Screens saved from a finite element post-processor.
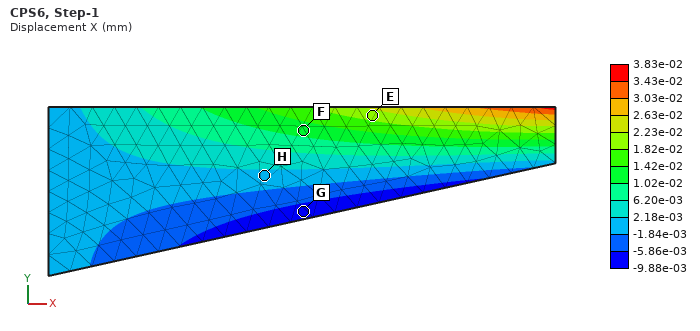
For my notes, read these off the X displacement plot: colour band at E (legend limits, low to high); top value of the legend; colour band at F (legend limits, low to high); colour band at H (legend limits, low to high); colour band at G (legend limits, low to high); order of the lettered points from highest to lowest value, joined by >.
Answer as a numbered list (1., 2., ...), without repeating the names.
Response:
1. 1.82e-02 to 2.23e-02 mm
2. 3.83e-02 mm
3. 1.02e-02 to 1.42e-02 mm
4. -1.84e-03 to 2.18e-03 mm
5. -9.88e-03 to -5.86e-03 mm
6. E > F > H > G
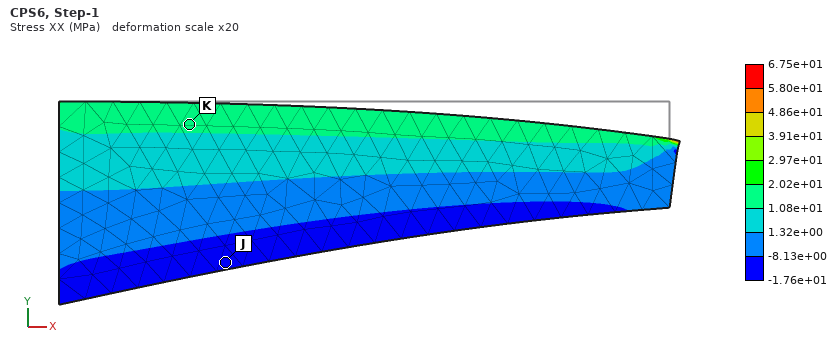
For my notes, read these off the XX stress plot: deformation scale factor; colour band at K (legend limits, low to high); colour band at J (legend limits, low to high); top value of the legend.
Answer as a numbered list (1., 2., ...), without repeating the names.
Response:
1. 20
2. 1.08e+01 to 2.02e+01 MPa
3. -1.76e+01 to -8.13e+00 MPa
4. 6.75e+01 MPa
